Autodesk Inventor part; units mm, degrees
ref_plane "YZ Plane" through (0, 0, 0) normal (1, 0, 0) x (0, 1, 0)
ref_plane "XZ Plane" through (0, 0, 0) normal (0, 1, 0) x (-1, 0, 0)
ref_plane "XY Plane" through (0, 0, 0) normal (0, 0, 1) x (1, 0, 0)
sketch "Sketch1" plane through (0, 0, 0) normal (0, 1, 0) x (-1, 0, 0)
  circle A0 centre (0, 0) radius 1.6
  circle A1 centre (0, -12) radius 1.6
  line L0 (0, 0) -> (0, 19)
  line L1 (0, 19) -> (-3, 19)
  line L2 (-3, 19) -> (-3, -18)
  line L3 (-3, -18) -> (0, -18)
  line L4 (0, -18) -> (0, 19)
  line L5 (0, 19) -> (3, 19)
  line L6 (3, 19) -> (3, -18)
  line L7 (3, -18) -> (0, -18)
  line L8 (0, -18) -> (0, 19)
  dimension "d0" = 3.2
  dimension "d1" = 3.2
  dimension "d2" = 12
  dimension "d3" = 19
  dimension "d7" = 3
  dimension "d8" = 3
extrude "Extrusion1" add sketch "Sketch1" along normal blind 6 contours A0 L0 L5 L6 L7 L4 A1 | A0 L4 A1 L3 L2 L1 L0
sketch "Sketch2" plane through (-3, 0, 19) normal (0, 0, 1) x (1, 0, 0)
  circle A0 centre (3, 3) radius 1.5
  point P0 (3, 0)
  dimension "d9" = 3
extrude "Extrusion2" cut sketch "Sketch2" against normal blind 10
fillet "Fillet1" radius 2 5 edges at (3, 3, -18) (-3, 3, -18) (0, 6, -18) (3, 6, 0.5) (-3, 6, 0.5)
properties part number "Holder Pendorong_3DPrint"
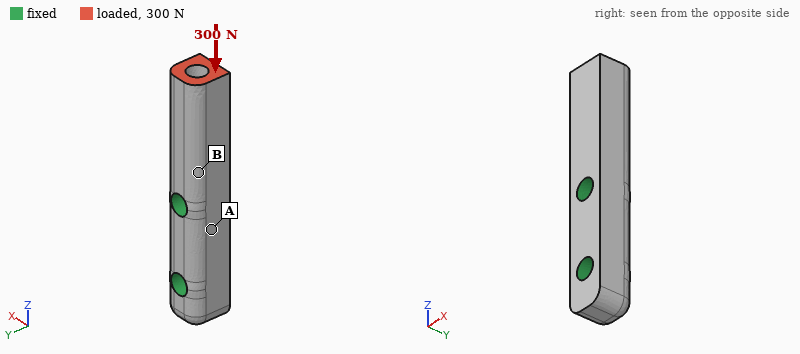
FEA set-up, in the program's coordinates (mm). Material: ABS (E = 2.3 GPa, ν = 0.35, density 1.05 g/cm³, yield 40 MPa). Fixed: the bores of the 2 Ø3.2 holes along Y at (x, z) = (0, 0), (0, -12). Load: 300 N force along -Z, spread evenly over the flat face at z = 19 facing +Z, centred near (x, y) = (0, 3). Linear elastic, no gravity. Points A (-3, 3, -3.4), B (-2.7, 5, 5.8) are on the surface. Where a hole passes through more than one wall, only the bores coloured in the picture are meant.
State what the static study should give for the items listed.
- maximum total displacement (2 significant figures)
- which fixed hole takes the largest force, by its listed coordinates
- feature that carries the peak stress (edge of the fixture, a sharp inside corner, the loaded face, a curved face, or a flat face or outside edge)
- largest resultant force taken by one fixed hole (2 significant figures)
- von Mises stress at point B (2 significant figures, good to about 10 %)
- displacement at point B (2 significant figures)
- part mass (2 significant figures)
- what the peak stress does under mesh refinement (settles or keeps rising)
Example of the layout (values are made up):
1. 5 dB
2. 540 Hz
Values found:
1. 83 µm
2. (0, 0)
3. edge of the fixture
4. 300 N
5. 8.8 MPa
6. 19 µm
7. 1.1 g
8. keeps rising
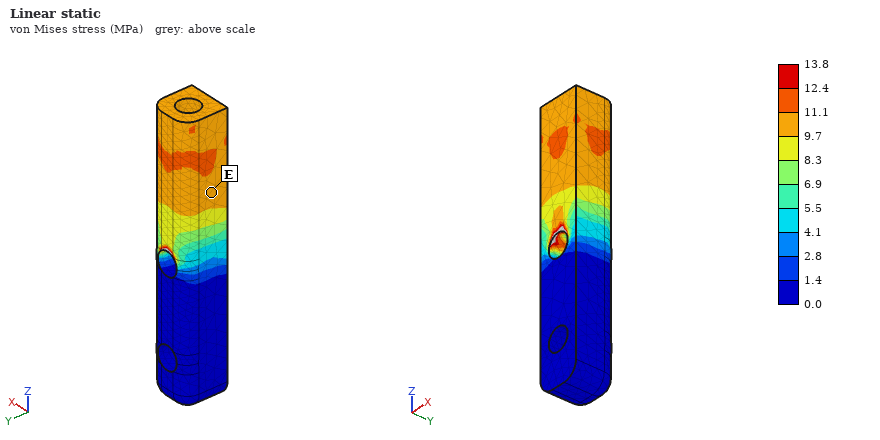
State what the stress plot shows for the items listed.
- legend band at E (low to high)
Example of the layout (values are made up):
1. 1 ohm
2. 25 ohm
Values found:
1. 9.7 to 11.1 MPa
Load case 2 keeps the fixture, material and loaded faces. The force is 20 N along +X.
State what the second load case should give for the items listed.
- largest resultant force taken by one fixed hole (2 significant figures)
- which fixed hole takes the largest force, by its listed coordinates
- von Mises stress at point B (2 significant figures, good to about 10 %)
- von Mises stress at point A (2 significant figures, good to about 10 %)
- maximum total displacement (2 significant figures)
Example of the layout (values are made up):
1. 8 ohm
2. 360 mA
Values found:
1. 24 N
2. (0, 0)
3. 7.5 MPa
4. 0.90 MPa
5. 0.23 mm
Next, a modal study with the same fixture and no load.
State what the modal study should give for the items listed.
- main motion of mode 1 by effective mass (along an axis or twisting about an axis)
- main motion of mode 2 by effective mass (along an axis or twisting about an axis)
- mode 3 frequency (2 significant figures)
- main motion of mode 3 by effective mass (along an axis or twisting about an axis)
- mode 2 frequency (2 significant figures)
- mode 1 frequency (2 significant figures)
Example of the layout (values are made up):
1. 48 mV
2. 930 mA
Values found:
1. along X
2. along Y
3. 12 kHz
4. twisting about Z
5. 4400 Hz
6. 4000 Hz
